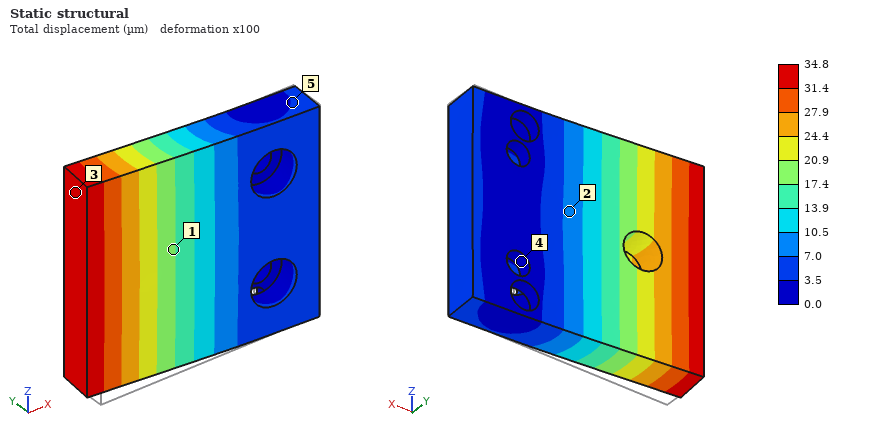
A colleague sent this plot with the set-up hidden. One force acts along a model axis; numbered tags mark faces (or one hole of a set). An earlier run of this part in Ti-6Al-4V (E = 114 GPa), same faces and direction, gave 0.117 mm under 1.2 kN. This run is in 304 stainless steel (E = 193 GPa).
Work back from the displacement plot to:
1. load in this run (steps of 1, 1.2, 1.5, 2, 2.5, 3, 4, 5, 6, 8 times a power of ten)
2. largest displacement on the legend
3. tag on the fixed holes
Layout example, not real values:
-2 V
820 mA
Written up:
600 N
34.8 µm
4
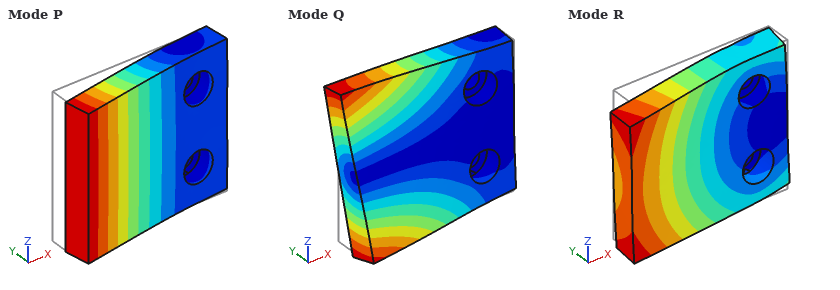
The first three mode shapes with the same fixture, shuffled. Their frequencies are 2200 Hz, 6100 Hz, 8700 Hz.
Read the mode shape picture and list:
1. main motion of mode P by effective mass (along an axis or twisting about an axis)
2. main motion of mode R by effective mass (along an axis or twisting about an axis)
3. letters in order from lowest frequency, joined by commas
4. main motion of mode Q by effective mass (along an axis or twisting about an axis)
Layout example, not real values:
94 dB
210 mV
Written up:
along Y
along Z
P, Q, R
twisting about X
